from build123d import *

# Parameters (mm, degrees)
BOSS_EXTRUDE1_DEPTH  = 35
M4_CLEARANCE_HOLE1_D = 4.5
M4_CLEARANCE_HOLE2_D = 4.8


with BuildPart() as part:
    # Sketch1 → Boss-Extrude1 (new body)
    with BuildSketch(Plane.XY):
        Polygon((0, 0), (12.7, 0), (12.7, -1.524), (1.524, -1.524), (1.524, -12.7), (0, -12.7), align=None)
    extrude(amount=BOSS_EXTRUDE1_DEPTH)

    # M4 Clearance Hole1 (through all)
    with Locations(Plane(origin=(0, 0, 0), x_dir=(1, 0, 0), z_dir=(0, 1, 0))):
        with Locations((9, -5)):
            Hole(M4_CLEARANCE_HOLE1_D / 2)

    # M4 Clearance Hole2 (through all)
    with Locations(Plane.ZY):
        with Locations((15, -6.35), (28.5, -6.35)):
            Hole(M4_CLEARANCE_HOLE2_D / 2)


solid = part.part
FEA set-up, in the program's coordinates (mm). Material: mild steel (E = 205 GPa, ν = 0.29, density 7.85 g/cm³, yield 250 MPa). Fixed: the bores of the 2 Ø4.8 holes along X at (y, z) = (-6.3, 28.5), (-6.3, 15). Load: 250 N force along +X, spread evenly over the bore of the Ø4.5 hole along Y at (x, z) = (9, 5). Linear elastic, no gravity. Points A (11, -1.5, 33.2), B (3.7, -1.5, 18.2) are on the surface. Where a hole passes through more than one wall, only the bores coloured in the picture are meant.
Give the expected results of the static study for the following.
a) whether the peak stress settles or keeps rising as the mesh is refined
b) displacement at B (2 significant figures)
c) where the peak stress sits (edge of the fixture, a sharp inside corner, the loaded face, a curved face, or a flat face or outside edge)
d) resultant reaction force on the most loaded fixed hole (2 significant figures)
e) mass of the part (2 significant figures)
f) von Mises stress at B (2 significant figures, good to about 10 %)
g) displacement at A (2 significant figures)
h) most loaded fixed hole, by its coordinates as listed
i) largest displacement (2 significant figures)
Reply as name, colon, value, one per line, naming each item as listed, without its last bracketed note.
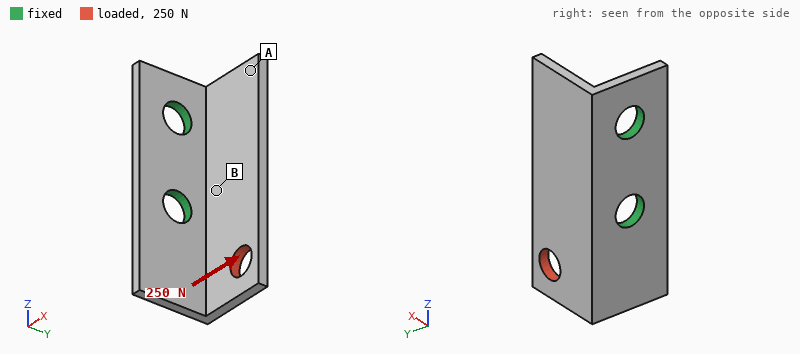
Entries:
whether the peak stress settles or keeps rising as the mesh is refined: keeps rising
displacement at B: 7.5 µm
where the peak stress sits: edge of the fixture
resultant reaction force on the most loaded fixed hole: 390 N
mass of the part: 9.4 g
von Mises stress at B: 49 MPa
displacement at A: 11 µm
most loaded fixed hole, by its coordinates as listed: (-6.3, 15)
largest displacement: 45 µm
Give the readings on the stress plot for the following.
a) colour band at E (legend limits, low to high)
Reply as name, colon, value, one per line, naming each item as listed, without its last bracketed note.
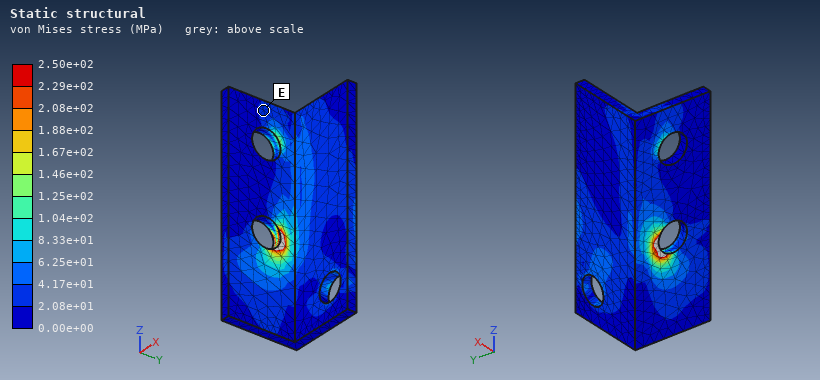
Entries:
colour band at E: 2.08e+01 to 4.17e+01 MPa
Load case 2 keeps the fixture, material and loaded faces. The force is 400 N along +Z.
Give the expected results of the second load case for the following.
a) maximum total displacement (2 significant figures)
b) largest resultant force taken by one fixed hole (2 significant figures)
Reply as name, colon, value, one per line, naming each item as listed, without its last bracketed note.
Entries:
maximum total displacement: 27 µm
largest resultant force taken by one fixed hole: 300 N
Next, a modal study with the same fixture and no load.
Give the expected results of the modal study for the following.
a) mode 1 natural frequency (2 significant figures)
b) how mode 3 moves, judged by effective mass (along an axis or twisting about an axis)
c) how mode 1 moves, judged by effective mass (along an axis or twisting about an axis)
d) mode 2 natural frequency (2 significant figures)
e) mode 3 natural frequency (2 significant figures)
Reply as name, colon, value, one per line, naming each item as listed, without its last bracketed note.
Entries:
mode 1 natural frequency: 5700 Hz
how mode 3 moves, judged by effective mass: along X
how mode 1 moves, judged by effective mass: along Y
mode 2 natural frequency: 8100 Hz
mode 3 natural frequency: 11 kHz
